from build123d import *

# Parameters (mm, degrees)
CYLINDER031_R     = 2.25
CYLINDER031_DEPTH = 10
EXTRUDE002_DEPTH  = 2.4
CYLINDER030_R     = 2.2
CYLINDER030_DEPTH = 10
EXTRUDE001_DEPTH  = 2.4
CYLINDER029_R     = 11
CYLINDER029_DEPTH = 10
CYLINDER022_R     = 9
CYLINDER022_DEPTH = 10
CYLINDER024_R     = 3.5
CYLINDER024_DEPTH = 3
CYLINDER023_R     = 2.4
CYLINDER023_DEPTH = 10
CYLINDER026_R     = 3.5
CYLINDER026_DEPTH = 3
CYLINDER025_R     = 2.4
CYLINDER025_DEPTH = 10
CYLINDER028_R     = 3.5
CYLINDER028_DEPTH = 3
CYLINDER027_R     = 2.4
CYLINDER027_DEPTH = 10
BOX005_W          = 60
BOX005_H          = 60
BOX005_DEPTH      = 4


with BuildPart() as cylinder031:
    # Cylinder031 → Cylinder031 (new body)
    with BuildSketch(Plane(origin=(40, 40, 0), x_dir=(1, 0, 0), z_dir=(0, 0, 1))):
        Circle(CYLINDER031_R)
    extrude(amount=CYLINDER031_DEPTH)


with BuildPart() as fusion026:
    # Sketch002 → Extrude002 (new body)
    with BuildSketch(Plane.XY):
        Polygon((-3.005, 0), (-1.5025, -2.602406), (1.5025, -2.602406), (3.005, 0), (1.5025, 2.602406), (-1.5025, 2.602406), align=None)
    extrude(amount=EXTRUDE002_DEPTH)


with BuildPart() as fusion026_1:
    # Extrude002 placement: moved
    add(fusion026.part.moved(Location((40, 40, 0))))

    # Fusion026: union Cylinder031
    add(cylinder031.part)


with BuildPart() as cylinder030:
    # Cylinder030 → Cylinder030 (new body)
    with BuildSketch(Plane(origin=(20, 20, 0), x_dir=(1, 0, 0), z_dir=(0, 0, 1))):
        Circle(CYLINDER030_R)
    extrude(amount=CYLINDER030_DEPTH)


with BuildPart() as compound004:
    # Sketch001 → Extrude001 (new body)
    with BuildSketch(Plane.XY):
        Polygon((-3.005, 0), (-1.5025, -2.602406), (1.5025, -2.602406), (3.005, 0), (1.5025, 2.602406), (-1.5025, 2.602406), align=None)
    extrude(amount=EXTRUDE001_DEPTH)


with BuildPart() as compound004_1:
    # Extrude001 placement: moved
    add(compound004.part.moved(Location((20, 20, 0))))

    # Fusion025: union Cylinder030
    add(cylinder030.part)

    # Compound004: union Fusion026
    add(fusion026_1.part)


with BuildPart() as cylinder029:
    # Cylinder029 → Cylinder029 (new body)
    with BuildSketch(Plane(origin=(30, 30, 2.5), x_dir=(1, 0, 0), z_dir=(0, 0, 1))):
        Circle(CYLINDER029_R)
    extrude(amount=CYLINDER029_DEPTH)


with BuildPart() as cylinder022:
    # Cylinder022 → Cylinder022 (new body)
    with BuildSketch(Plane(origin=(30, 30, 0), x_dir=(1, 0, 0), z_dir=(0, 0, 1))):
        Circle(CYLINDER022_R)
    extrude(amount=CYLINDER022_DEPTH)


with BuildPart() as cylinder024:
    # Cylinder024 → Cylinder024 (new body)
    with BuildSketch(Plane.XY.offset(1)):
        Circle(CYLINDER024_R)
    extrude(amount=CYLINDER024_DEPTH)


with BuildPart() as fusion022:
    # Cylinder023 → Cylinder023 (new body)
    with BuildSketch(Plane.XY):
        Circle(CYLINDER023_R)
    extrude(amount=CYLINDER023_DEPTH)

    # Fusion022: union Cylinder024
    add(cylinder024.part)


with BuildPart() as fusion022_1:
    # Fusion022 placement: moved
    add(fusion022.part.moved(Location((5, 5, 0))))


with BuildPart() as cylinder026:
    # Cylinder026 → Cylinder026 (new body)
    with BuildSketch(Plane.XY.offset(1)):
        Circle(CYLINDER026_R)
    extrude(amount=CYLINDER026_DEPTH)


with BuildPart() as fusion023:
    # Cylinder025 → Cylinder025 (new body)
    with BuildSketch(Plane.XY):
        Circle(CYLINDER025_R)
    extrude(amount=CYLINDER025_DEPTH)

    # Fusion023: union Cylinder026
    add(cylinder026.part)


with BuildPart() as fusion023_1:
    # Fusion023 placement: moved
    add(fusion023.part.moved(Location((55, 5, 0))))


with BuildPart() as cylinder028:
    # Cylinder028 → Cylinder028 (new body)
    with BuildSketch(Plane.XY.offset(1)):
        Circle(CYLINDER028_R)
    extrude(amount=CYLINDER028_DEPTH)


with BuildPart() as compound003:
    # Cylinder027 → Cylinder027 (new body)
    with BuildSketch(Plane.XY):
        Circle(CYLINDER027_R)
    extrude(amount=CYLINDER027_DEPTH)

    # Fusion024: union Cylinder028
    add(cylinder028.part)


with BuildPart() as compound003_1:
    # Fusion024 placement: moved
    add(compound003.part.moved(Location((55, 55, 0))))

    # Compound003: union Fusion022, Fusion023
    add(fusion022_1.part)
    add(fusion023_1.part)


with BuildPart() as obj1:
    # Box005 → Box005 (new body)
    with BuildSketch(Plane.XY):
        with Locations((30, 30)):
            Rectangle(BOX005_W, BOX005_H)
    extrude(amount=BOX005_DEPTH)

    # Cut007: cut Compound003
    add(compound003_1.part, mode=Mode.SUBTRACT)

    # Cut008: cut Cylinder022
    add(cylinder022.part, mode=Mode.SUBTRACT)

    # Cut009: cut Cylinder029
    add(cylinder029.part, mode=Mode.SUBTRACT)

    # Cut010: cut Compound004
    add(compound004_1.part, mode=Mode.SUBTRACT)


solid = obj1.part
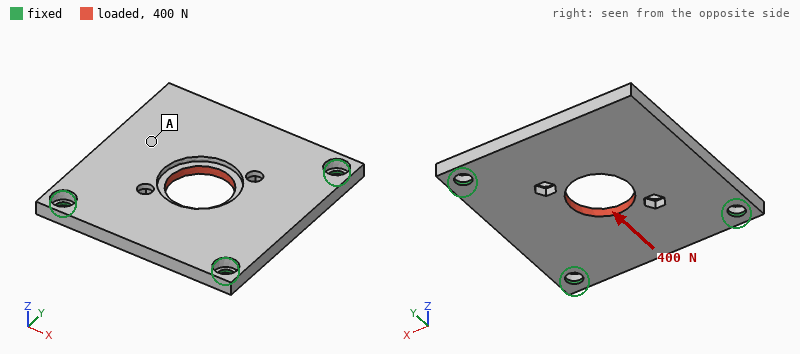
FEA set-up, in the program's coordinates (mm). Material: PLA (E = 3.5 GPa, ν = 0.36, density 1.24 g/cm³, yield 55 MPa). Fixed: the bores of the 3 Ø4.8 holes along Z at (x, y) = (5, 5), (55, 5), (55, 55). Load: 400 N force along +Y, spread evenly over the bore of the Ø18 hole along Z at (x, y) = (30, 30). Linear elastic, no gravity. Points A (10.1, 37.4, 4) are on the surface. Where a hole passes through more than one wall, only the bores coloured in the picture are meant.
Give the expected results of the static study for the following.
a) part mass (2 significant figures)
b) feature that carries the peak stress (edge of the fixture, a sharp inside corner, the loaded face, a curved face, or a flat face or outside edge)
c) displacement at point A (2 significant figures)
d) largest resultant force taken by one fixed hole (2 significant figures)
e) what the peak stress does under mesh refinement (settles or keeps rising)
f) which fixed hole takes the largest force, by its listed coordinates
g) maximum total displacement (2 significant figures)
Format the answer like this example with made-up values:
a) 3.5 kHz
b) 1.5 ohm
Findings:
a) 16 g
b) edge of the fixture
c) 41 µm
d) 160 N
e) keeps rising
f) (5, 5)
g) 59 µm
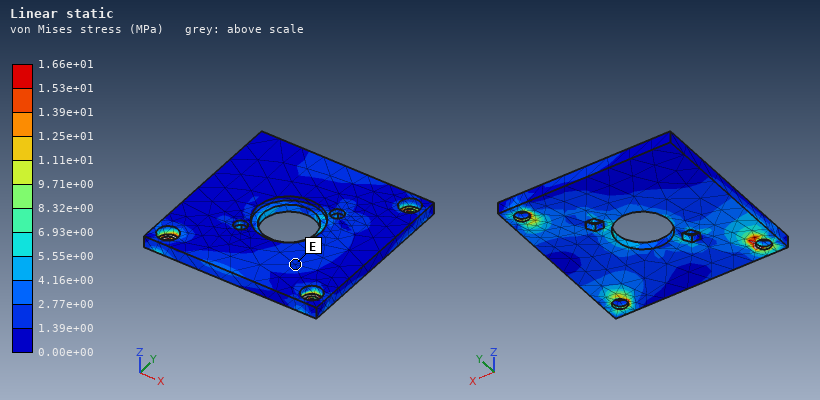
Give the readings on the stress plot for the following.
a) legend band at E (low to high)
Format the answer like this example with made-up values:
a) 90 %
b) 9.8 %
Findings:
a) 1.39e+00 to 2.77e+00 MPa
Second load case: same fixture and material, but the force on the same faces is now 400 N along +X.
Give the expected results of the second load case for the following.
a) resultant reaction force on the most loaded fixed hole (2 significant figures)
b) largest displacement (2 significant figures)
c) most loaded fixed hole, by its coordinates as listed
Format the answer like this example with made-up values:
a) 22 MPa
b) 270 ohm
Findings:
a) 160 N
b) 59 µm
c) (55, 55)
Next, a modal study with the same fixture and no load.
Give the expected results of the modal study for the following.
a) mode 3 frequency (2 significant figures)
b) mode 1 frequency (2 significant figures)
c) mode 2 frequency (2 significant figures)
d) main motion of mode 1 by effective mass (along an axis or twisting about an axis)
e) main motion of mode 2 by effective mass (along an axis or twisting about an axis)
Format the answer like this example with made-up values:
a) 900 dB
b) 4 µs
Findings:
a) 1900 Hz
b) 530 Hz
c) 1600 Hz
d) along Z
e) along Z
